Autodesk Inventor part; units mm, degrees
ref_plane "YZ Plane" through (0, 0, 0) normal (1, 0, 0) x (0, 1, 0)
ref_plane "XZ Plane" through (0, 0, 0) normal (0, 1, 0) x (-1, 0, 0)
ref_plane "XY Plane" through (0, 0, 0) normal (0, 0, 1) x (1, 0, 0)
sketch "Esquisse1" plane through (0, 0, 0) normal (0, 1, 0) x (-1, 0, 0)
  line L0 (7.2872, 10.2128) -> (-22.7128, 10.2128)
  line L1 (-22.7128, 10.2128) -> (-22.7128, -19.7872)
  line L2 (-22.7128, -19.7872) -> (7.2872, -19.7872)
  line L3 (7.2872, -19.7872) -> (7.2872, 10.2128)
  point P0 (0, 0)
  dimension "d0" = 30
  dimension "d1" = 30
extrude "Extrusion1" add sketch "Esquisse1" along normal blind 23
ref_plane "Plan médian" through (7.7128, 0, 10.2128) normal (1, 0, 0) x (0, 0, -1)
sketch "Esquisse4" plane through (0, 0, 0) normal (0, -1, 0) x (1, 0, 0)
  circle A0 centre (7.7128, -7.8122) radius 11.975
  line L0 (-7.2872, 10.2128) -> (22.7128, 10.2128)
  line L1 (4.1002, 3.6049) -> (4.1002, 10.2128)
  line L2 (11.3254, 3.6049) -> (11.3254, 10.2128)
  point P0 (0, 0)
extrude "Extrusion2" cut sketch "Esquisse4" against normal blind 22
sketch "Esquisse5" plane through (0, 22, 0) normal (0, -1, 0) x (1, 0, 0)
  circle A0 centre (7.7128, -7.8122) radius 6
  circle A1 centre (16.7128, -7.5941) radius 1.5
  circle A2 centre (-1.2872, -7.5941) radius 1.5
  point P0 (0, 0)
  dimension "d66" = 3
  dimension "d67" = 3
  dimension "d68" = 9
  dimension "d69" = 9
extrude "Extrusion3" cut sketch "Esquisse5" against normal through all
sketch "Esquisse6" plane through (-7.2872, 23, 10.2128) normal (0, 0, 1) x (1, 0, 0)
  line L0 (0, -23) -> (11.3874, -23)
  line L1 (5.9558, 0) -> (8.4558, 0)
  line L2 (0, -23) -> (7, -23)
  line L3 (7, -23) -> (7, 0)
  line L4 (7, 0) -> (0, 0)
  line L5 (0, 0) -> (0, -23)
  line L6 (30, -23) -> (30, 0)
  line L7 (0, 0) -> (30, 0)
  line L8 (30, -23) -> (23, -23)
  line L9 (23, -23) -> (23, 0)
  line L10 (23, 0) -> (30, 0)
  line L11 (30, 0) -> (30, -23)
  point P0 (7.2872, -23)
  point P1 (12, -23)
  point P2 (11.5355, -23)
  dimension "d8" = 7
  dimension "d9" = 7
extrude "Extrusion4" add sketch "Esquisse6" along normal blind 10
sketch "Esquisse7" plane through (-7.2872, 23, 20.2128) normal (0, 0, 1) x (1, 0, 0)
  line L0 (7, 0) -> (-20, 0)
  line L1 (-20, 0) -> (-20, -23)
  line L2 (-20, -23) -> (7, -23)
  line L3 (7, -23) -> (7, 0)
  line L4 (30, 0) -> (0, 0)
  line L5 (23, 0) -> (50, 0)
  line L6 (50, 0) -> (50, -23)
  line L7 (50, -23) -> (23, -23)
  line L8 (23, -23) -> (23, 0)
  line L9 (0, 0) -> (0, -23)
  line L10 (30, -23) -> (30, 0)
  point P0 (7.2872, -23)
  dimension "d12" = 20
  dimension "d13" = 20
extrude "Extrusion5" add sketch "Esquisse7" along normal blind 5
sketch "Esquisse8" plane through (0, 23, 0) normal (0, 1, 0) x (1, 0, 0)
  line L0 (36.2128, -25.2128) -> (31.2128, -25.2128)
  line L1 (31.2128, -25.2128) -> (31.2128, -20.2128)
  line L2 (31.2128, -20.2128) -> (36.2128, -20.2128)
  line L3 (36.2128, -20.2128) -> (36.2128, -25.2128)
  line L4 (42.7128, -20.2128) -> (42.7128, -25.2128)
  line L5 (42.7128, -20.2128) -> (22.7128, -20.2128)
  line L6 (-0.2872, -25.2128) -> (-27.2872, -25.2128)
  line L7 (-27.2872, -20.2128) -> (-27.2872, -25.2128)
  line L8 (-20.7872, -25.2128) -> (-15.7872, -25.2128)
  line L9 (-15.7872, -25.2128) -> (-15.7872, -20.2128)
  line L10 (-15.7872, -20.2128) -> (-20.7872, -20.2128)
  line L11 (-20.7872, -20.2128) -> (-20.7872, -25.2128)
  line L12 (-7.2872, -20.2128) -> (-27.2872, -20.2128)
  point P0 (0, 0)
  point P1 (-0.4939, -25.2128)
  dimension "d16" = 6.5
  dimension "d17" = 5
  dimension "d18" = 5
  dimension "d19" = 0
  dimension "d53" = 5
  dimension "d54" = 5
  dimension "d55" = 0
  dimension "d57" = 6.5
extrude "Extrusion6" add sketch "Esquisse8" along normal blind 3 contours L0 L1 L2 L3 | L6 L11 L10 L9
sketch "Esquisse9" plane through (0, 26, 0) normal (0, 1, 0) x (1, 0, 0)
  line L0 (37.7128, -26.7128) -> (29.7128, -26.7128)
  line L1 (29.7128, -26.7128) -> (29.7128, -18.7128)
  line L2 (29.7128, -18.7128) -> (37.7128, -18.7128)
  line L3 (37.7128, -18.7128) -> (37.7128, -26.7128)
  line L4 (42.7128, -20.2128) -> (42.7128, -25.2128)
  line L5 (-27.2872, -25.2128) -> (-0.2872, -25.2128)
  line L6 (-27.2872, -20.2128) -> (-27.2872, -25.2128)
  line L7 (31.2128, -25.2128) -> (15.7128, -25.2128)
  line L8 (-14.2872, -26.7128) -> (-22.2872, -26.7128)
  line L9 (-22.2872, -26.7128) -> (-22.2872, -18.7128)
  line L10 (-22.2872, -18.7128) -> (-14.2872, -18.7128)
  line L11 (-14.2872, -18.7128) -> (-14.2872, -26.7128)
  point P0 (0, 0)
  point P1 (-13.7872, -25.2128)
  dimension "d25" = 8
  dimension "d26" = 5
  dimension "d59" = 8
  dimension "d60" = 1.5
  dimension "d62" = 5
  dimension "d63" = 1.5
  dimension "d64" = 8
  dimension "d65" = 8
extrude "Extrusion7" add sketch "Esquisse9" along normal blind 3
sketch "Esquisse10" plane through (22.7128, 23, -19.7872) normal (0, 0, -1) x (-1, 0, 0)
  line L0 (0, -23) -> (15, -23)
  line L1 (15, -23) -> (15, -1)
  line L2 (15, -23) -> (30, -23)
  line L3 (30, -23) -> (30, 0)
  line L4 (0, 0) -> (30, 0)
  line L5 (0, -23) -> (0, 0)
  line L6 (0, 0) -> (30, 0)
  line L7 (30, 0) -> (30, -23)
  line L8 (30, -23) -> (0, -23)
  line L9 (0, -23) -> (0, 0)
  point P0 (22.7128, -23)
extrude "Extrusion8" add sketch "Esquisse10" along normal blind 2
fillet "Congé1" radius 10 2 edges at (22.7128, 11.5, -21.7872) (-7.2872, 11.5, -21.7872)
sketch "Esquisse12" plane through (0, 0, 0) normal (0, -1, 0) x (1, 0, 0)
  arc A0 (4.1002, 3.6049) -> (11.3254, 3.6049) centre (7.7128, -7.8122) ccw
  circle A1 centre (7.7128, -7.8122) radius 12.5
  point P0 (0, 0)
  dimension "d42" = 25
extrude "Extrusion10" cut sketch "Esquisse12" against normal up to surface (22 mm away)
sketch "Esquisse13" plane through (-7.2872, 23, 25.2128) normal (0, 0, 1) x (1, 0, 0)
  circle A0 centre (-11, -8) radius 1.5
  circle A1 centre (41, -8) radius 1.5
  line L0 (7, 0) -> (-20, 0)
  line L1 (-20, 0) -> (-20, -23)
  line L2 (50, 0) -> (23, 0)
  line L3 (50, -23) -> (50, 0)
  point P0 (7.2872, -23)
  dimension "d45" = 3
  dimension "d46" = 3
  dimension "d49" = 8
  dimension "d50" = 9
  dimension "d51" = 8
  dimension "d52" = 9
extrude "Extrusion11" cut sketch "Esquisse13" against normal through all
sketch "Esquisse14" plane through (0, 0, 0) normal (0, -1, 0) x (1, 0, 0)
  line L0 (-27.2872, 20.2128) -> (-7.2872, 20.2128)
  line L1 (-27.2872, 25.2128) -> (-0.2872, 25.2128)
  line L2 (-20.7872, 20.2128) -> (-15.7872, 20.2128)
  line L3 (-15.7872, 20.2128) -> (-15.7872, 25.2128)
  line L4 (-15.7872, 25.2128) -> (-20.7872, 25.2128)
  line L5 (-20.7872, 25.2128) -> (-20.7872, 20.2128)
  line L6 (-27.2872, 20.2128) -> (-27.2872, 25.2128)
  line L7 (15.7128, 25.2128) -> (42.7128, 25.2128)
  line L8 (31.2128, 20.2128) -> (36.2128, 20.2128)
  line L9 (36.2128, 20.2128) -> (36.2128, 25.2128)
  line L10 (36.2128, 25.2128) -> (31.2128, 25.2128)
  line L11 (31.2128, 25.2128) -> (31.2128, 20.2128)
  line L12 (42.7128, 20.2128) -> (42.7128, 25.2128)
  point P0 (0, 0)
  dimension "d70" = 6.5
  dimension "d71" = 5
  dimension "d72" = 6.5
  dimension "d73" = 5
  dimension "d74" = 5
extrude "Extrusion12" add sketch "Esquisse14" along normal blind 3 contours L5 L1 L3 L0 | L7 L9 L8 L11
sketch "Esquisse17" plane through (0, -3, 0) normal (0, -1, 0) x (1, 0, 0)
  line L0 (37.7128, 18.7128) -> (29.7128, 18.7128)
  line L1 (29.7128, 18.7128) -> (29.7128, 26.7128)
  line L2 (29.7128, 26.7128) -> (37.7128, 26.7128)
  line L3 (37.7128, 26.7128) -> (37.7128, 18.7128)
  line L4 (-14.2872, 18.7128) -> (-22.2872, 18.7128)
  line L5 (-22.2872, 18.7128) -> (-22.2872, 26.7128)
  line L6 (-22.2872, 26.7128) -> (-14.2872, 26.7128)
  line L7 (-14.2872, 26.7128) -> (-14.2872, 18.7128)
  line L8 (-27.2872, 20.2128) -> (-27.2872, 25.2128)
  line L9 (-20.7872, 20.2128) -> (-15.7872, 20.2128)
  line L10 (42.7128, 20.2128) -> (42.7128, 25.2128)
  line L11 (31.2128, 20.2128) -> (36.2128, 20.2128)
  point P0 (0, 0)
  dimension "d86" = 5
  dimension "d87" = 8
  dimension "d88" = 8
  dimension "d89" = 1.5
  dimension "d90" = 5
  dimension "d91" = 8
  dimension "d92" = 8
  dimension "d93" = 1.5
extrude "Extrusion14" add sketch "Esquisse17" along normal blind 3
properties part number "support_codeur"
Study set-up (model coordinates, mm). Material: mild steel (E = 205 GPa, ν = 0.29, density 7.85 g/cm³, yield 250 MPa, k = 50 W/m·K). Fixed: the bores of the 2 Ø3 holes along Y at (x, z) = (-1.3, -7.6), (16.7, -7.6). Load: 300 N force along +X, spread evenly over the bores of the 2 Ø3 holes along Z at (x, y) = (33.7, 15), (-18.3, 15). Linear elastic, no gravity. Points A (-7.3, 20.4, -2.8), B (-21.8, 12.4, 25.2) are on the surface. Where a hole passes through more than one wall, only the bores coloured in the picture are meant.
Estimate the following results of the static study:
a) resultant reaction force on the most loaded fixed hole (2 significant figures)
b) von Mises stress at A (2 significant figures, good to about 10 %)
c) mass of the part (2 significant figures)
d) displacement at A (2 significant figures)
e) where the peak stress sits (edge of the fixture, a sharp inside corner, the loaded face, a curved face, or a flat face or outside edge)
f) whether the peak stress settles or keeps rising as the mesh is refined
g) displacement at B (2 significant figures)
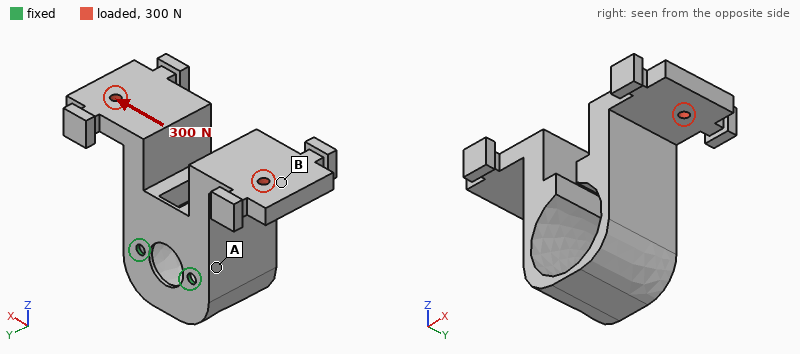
460 N
14 MPa
150 g
5.7 µm
edge of the fixture
keeps rising
28 µm
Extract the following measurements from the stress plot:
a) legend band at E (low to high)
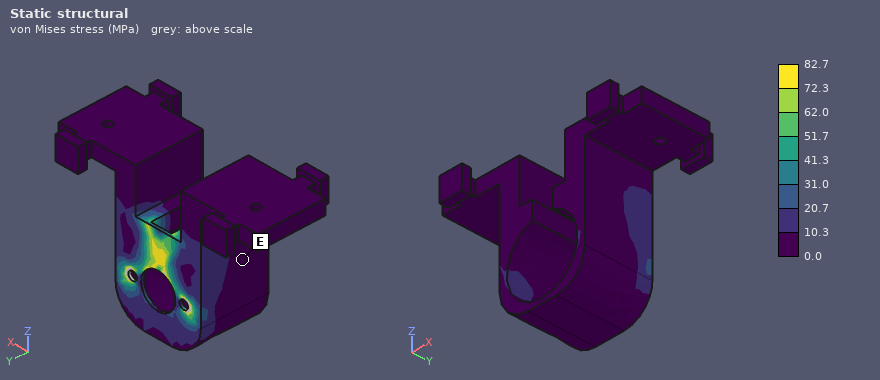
0.0 to 10.3 MPa
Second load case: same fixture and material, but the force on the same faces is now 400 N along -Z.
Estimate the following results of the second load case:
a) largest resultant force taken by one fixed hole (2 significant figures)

230 N
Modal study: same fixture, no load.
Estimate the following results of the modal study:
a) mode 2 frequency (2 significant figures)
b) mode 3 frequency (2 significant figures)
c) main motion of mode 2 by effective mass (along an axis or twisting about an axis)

1400 Hz
1600 Hz
along X
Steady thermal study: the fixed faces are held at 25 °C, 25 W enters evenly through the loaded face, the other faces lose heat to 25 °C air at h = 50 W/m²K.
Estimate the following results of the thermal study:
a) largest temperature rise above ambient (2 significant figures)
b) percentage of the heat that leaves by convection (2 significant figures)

72 K
75 %
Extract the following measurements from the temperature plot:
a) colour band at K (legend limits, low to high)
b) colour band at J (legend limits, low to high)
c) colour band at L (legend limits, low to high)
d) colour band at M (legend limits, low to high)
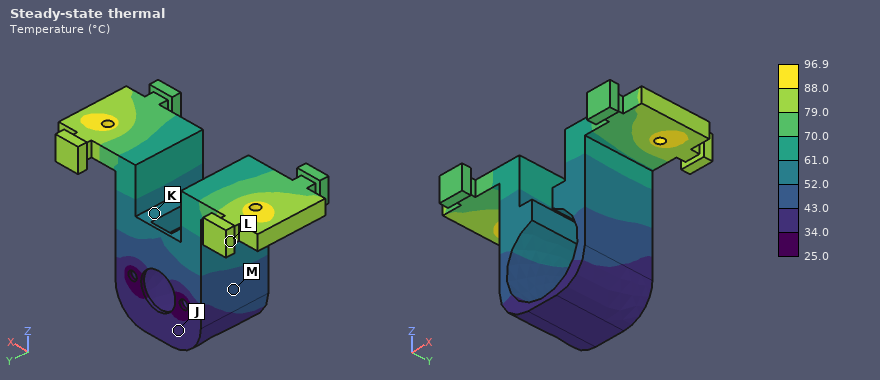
52.0 to 61.0 °C
34.0 to 43.0 °C
79.0 to 88.0 °C
43.0 to 52.0 °C
